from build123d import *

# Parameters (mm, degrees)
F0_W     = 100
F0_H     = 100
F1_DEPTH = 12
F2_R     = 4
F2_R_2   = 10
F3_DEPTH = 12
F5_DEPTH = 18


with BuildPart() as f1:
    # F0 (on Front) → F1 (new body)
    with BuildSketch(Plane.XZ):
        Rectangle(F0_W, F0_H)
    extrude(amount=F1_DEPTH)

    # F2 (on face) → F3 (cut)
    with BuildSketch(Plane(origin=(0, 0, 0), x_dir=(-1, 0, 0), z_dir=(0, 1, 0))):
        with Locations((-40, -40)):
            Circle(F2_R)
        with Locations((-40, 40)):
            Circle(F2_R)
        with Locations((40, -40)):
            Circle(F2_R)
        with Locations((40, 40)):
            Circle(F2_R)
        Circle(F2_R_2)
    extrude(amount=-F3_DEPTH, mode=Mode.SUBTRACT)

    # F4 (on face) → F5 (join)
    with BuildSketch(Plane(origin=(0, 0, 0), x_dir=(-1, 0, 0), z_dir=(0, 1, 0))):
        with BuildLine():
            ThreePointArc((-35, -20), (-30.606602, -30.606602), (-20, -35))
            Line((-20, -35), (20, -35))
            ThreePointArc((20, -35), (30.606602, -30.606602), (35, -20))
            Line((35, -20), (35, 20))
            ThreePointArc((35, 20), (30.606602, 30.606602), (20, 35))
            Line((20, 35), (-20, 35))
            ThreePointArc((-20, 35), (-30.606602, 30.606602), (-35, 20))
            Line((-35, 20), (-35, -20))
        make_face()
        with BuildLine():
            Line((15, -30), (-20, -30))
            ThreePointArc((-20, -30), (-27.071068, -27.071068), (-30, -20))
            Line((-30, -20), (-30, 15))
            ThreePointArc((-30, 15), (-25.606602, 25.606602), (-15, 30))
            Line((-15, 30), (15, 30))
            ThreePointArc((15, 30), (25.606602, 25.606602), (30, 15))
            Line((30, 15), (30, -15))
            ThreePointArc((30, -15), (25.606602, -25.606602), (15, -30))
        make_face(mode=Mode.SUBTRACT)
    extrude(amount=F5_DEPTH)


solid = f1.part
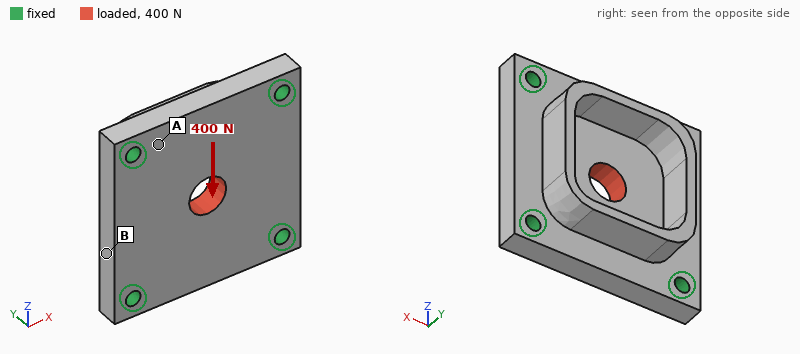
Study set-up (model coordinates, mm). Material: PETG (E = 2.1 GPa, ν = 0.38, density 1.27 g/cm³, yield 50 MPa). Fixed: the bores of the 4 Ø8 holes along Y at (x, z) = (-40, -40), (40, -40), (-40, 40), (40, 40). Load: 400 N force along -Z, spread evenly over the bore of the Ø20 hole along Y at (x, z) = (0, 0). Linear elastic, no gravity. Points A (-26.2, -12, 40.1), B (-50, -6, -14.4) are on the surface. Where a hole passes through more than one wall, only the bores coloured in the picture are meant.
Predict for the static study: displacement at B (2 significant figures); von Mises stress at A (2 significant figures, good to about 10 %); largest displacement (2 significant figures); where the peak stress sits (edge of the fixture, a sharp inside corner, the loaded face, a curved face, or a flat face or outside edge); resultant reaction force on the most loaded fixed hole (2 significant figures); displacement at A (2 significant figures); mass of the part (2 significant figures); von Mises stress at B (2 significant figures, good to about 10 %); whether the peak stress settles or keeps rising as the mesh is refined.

2.0 µm
0.27 MPa
12 µm
edge of the fixture
110 N
4.2 µm
170 g
0.082 MPa
keeps rising
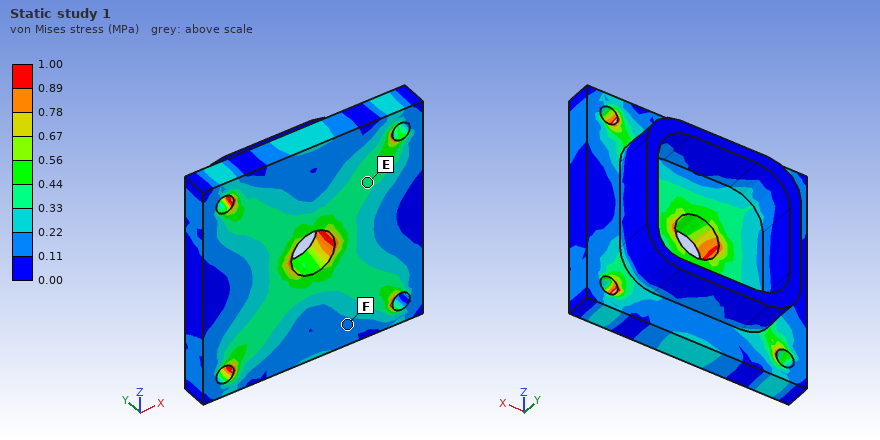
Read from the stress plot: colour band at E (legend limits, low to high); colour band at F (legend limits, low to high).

0.33 to 0.44 MPa
0.11 to 0.22 MPa
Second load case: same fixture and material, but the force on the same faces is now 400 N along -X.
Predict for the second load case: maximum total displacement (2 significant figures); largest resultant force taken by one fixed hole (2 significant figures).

12 µm
110 N
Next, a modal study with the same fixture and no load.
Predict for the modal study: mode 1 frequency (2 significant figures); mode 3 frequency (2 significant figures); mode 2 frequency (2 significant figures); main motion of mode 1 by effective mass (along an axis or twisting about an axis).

1700 Hz
2500 Hz
2500 Hz
along Y
